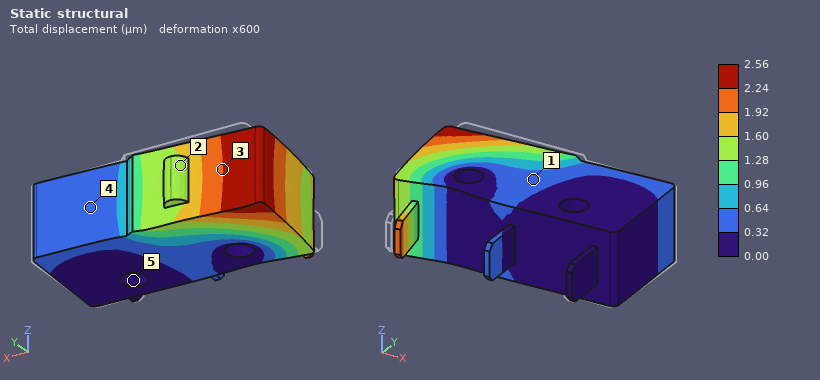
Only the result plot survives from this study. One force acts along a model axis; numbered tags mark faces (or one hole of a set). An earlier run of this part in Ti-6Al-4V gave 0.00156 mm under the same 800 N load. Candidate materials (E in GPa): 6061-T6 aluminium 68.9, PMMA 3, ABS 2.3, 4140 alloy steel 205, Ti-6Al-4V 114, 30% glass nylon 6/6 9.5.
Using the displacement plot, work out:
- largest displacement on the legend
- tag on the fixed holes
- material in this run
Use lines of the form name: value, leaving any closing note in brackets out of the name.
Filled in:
largest displacement on the legend: 2.56 µm
tag on the fixed holes: 5
material in this run: 6061-T6 aluminium
